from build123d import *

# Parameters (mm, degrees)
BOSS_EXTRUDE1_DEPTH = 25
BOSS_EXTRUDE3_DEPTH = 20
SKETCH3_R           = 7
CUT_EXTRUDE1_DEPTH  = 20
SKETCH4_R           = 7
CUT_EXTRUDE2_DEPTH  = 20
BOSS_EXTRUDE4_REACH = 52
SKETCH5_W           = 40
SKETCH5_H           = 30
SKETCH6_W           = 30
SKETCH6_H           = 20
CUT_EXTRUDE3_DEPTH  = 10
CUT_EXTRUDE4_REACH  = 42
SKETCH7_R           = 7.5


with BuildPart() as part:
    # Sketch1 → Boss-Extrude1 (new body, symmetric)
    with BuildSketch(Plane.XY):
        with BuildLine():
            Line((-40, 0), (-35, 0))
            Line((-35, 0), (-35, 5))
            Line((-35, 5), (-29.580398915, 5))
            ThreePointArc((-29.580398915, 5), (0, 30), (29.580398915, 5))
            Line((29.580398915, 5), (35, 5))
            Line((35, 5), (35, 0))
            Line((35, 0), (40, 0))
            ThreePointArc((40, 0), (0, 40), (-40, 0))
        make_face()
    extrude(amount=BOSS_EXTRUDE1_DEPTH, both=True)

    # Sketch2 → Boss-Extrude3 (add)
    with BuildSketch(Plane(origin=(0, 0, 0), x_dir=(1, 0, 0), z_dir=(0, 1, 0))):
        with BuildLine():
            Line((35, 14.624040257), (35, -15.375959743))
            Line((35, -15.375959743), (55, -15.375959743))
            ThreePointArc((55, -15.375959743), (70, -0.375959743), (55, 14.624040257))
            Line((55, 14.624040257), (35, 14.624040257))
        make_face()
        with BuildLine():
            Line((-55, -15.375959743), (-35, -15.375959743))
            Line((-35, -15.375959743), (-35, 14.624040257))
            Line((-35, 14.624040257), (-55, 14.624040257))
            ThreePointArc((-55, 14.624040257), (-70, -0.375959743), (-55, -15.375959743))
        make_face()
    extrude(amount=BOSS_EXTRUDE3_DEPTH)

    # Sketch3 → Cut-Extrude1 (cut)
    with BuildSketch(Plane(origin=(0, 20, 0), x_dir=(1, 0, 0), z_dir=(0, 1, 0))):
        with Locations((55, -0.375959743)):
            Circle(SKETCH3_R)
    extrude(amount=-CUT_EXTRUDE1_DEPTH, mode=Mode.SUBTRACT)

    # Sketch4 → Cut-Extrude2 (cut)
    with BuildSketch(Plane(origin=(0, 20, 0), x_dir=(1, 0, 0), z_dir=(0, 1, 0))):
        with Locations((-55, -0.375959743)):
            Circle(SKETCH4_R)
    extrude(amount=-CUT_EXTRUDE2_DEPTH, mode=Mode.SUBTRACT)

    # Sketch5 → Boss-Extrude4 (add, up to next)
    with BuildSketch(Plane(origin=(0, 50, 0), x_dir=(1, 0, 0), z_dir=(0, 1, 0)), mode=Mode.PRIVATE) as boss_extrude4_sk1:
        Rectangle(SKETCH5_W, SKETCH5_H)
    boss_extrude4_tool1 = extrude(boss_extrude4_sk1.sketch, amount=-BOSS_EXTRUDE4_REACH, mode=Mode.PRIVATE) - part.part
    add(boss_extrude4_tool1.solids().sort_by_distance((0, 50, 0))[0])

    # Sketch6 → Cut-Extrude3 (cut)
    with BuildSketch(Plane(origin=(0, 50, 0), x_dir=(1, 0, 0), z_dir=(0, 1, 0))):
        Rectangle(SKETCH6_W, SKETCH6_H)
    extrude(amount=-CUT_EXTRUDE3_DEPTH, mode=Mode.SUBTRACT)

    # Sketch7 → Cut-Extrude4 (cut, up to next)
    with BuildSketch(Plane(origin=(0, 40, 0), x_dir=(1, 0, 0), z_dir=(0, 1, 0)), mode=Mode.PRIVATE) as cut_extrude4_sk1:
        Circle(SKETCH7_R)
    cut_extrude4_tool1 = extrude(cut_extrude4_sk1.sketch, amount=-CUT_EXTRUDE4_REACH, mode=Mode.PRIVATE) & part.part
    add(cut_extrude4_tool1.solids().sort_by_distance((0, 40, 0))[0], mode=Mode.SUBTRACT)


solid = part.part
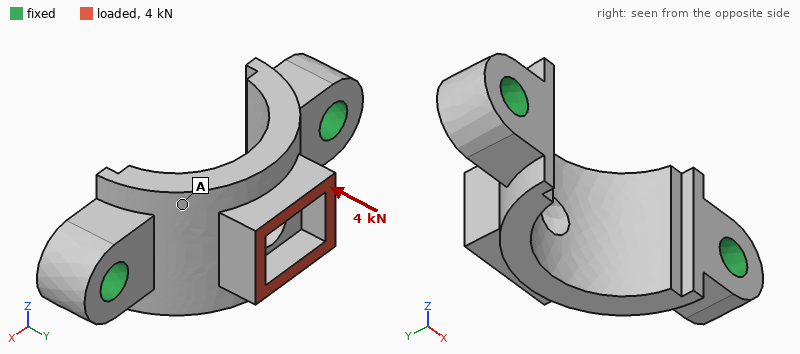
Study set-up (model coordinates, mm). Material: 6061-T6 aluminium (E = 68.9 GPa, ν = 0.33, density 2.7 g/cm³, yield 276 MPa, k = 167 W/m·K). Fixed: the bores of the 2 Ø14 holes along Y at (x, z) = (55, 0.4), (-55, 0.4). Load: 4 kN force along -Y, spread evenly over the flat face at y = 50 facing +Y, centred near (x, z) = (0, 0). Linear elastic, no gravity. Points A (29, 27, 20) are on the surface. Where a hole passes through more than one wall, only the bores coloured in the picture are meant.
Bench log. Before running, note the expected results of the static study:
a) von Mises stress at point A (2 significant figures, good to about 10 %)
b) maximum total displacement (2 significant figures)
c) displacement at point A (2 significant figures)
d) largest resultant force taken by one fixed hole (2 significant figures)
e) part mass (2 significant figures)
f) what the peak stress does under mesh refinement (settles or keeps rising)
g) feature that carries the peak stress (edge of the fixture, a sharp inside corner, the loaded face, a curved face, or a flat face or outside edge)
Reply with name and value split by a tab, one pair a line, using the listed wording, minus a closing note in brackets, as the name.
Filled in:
von Mises stress at point A	3.1 MPa
maximum total displacement	11 µm
displacement at point A	5.3 µm
largest resultant force taken by one fixed hole	2.7 kN
part mass	230 g
what the peak stress does under mesh refinement	keeps rising
feature that carries the peak stress	edge of the fixture
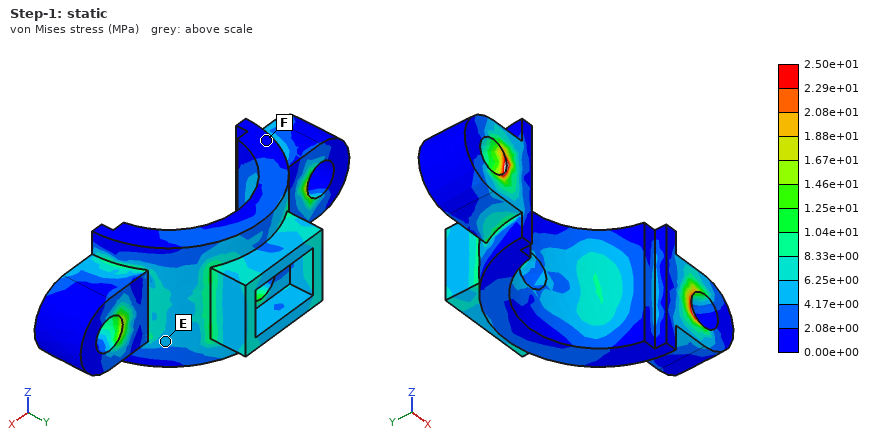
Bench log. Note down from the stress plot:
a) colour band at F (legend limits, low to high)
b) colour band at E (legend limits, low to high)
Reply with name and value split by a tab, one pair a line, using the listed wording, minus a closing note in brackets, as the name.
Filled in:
colour band at F	0.00e+00 to 2.08e+00 MPa
colour band at E	4.17e+00 to 6.25e+00 MPa
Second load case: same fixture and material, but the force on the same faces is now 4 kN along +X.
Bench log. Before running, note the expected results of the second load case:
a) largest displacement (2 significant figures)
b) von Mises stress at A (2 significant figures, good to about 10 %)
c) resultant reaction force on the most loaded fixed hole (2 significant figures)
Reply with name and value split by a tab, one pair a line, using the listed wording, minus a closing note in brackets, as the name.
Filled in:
largest displacement	26 µm
von Mises stress at A	5.2 MPa
resultant reaction force on the most loaded fixed hole	2.8 kN
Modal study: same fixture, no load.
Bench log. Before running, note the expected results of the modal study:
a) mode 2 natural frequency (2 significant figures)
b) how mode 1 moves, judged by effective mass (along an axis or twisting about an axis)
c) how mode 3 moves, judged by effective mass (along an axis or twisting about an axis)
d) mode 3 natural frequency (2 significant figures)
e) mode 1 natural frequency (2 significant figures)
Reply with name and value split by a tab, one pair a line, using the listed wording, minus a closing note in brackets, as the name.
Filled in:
mode 2 natural frequency	9900 Hz
how mode 1 moves, judged by effective mass	along Z
how mode 3 moves, judged by effective mass	along X
mode 3 natural frequency	10 kHz
mode 1 natural frequency	4700 Hz
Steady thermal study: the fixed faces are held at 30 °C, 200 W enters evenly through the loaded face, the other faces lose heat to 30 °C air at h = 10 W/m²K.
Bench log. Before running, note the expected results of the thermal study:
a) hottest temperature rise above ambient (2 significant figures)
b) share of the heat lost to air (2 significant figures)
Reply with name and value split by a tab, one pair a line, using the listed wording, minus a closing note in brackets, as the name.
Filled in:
hottest temperature rise above ambient	79 K
share of the heat lost to air	3.2 %
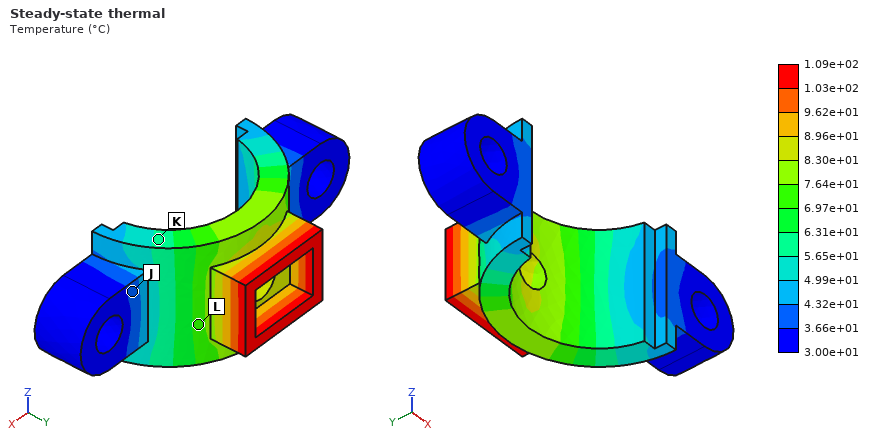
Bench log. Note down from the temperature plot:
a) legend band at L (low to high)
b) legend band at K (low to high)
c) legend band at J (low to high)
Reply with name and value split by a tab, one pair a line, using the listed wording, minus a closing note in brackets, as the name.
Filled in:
legend band at L	6.97e+01 to 7.64e+01 °C
legend band at K	5.65e+01 to 6.31e+01 °C
legend band at J	3.66e+01 to 4.32e+01 °C
